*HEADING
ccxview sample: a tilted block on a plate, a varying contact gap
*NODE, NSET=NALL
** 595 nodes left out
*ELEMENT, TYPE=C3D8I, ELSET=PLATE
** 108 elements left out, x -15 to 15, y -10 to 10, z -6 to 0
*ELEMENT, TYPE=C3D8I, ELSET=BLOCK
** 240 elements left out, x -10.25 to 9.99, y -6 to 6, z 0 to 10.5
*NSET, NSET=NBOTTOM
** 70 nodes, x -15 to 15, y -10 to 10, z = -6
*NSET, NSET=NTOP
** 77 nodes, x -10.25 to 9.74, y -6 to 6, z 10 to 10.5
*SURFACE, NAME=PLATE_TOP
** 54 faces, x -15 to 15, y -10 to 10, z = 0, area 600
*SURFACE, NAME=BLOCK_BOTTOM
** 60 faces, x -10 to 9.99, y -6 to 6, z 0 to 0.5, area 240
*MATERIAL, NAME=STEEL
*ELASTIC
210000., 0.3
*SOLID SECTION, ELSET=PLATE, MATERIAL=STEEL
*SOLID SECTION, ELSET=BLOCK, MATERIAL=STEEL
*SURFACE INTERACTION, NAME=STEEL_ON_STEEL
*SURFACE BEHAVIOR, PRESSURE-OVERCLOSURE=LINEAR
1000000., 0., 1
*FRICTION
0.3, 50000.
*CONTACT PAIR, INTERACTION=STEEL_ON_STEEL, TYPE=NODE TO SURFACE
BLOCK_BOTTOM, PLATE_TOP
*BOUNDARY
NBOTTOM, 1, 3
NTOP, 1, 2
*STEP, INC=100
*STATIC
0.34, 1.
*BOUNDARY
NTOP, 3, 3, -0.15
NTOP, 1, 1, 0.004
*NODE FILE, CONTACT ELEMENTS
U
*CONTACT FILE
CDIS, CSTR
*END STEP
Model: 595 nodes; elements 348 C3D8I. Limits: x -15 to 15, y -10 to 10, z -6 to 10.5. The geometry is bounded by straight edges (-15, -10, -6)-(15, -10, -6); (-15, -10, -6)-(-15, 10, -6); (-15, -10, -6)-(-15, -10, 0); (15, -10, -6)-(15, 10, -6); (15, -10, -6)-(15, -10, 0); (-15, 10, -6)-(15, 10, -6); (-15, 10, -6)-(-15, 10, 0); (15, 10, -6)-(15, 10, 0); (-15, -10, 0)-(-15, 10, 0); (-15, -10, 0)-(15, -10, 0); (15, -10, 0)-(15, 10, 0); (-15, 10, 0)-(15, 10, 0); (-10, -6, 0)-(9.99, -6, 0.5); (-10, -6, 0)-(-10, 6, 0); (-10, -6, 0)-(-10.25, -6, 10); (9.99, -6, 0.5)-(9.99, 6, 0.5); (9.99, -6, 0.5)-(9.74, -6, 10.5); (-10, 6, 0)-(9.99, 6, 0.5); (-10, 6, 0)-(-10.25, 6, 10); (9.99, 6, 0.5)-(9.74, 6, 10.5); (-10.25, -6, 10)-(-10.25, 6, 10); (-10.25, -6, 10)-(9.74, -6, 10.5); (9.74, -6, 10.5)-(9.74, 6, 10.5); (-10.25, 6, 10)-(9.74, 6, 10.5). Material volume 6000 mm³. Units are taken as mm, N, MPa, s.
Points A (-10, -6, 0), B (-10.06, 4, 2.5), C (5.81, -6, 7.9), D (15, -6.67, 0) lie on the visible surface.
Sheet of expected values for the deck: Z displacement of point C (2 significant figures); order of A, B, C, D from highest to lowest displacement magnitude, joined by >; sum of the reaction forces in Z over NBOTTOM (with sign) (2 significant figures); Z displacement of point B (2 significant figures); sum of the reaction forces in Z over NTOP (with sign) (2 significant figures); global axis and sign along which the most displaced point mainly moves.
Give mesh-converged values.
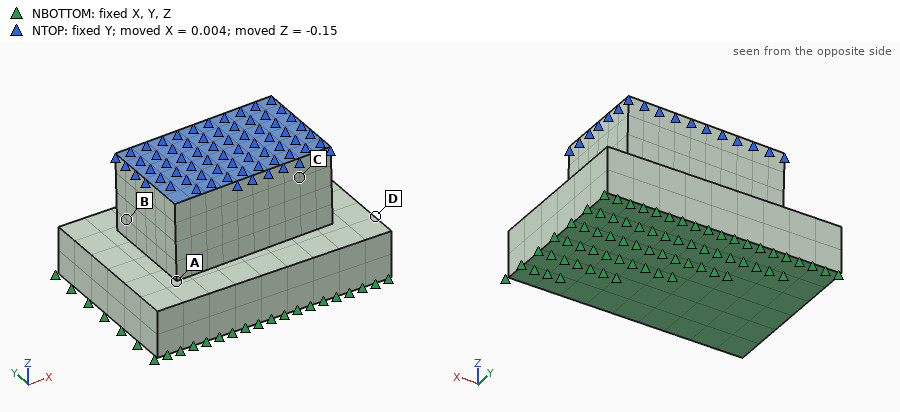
-0.15 mm
C > B > A > D
100000 N
-0.083 mm
-100000 N
-Z
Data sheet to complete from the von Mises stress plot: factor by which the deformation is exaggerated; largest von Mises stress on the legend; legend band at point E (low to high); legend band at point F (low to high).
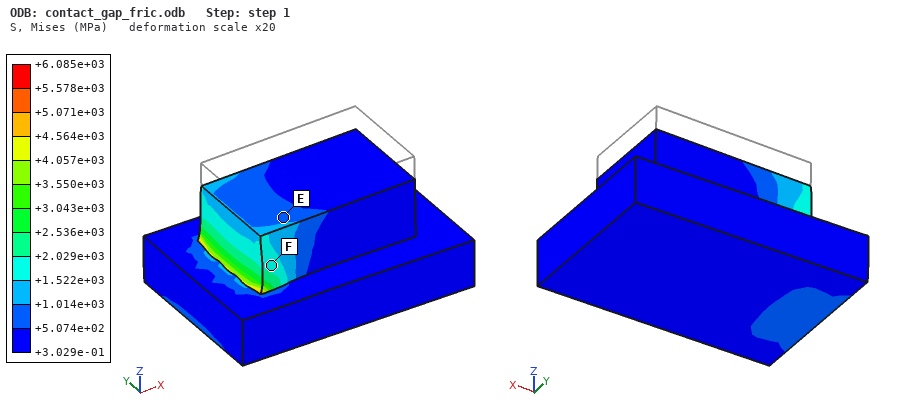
20
+6.085e+03 MPa
+5.074e+02 to +1.014e+03 MPa
+1.522e+03 to +2.029e+03 MPa
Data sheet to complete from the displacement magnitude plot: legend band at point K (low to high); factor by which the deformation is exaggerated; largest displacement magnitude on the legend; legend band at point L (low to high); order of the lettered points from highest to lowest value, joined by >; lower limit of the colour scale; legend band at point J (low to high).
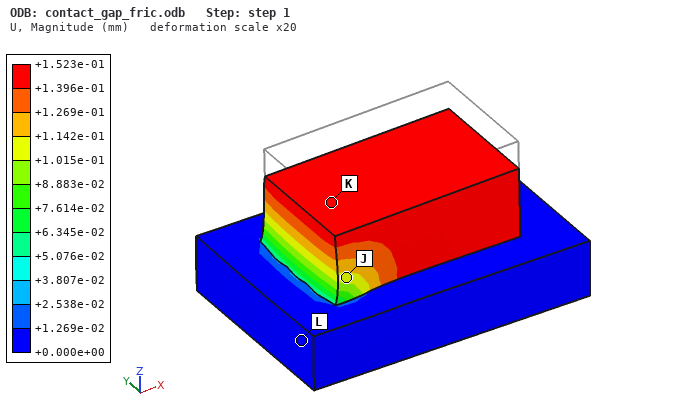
+1.396e-01 to +1.523e-01 mm
20
+1.523e-01 mm
+0.000e+00 to +1.269e-02 mm
K > J > L
+0.000e+00 mm
+1.015e-01 to +1.142e-01 mm
